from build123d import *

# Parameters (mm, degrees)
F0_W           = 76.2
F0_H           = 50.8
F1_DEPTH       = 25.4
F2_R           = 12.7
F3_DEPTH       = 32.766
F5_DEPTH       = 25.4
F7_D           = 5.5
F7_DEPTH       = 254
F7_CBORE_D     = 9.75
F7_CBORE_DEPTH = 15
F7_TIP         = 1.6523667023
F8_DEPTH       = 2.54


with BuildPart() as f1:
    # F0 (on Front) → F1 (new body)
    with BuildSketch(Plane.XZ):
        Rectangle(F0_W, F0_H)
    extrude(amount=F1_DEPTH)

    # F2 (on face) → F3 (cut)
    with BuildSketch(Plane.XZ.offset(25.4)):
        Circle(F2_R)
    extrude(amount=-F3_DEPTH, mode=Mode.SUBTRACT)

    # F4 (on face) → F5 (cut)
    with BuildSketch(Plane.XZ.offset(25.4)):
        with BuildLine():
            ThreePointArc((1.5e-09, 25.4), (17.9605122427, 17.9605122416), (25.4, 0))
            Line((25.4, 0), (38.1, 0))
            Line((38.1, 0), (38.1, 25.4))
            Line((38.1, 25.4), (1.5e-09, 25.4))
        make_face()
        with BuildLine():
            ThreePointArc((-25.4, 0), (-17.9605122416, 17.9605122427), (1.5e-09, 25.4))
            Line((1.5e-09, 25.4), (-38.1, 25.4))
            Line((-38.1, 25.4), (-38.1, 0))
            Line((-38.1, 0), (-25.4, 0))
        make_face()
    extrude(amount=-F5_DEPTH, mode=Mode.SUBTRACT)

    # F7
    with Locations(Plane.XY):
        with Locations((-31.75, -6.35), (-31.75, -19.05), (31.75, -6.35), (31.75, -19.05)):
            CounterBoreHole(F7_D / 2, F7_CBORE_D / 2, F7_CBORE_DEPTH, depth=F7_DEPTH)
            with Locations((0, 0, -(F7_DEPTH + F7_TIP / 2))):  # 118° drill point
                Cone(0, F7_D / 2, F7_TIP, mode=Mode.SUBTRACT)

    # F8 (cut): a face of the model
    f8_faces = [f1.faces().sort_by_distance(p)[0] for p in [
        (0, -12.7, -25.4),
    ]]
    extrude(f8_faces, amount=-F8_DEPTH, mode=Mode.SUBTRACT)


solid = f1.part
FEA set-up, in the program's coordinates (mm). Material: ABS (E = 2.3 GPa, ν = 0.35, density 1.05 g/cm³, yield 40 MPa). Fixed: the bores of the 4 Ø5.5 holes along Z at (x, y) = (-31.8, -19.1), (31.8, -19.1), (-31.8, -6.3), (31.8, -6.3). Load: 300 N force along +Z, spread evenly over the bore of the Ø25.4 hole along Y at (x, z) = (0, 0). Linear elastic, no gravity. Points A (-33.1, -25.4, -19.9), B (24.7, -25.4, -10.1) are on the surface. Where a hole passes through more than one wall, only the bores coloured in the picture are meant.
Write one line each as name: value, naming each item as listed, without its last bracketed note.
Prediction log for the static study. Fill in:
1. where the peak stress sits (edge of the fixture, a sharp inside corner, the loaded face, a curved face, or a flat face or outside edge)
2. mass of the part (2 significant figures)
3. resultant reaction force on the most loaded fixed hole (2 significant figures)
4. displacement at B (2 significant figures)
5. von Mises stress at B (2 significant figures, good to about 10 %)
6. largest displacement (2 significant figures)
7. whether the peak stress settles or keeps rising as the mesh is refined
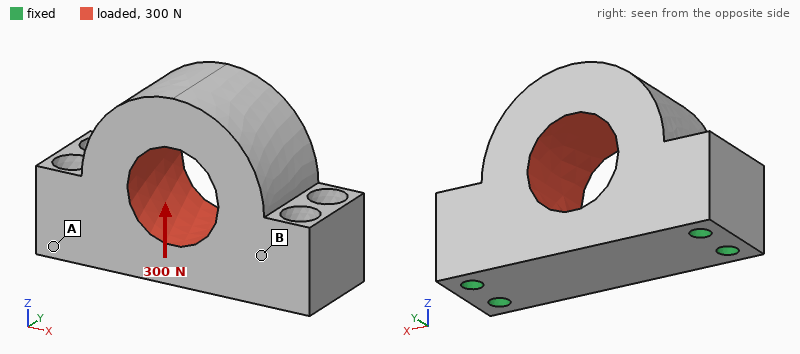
where the peak stress sits: edge of the fixture
mass of the part: 54 g
resultant reaction force on the most loaded fixed hole: 83 N
displacement at B: 7.5 µm
von Mises stress at B: 0.57 MPa
largest displacement: 18 µm
whether the peak stress settles or keeps rising as the mesh is refined: keeps rising
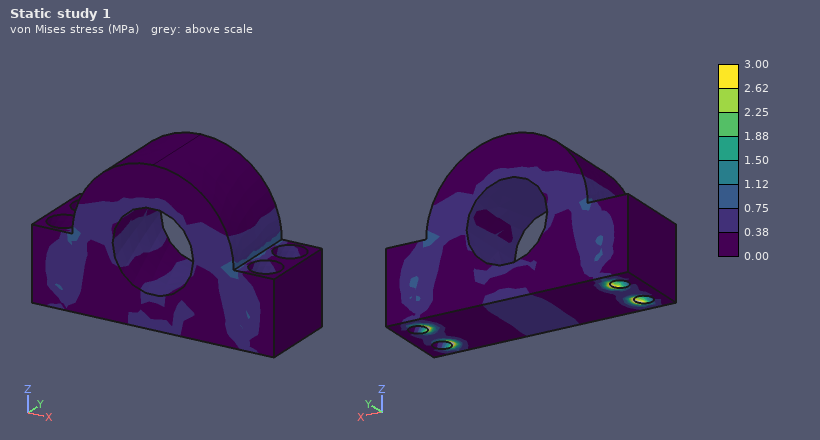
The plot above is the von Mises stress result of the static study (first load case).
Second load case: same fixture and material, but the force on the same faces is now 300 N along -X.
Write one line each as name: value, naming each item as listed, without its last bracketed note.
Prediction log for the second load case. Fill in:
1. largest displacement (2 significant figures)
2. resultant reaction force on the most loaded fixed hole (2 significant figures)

largest displacement: 19 µm
resultant reaction force on the most loaded fixed hole: 87 N
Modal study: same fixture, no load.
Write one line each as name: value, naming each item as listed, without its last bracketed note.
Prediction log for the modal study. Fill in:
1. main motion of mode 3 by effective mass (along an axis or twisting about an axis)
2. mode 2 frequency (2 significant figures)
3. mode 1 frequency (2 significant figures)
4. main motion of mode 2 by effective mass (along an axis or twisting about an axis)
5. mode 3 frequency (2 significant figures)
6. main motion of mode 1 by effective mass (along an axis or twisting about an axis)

main motion of mode 3 by effective mass: along Z
mode 2 frequency: 3500 Hz
mode 1 frequency: 1600 Hz
main motion of mode 2 by effective mass: along X
mode 3 frequency: 3800 Hz
main motion of mode 1 by effective mass: along Y
